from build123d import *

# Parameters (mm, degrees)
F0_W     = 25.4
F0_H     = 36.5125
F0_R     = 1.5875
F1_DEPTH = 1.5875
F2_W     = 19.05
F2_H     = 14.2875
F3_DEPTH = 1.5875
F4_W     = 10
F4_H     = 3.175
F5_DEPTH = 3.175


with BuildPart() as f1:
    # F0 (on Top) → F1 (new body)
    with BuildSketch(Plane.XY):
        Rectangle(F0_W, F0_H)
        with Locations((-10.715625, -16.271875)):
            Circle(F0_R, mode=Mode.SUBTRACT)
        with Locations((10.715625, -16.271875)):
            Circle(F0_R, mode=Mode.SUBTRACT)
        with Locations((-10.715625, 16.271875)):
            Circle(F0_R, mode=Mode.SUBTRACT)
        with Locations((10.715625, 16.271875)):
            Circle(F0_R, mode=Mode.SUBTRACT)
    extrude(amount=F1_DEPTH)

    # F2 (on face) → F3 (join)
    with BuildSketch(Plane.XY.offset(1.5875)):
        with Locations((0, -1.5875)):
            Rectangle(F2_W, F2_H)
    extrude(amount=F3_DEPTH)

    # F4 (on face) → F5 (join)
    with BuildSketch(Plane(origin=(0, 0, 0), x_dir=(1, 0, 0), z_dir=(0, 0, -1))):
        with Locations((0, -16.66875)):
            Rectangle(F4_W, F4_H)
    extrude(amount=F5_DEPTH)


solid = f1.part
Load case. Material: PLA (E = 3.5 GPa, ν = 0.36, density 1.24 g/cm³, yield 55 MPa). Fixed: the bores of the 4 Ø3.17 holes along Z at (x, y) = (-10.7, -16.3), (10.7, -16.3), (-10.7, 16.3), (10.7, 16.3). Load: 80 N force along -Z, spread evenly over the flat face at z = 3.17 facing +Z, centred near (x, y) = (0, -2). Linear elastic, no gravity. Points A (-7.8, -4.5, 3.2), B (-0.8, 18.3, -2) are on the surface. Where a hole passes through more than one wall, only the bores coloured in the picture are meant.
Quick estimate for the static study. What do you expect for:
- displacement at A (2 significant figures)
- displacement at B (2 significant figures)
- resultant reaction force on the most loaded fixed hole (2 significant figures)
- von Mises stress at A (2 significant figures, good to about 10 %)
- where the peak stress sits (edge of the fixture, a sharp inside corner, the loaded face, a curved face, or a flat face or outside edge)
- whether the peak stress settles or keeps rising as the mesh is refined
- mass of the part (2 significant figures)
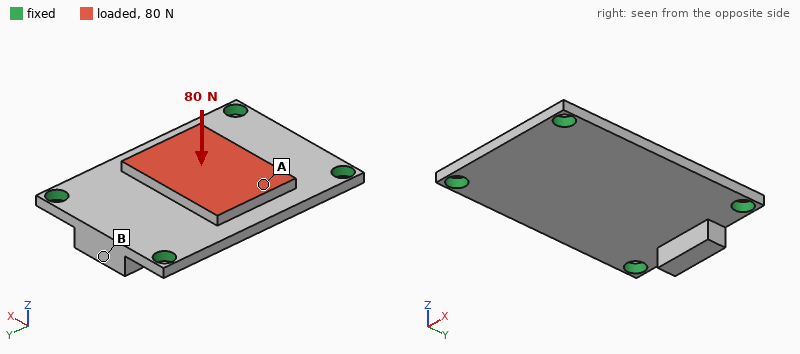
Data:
0.17 mm
0.052 mm
29 N
8.1 MPa
edge of the fixture
keeps rising
2.4 g
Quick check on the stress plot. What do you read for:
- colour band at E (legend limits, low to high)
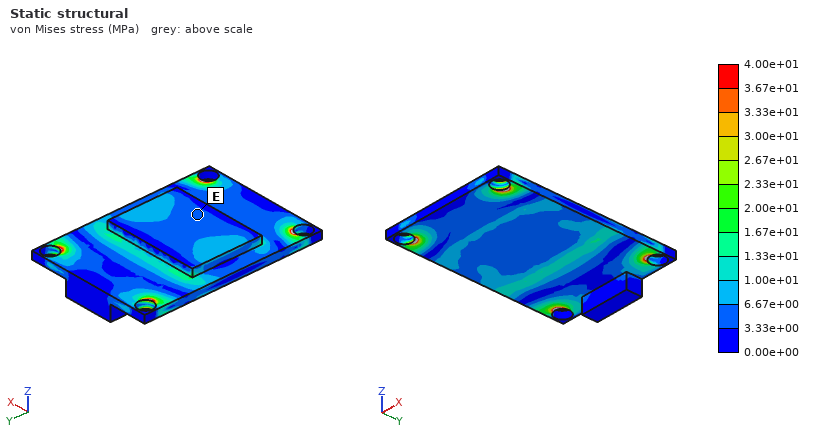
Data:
3.33e+00 to 6.67e+00 MPa
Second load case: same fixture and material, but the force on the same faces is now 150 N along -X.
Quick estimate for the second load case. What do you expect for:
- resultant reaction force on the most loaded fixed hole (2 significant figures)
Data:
56 N
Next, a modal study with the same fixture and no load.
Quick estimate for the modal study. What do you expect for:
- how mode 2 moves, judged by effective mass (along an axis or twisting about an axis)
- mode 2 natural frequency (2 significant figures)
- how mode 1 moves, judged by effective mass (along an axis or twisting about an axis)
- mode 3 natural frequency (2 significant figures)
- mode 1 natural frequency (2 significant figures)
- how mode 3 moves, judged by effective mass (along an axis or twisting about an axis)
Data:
twisting about Y
4000 Hz
along Z
6300 Hz
2700 Hz
twisting about X
